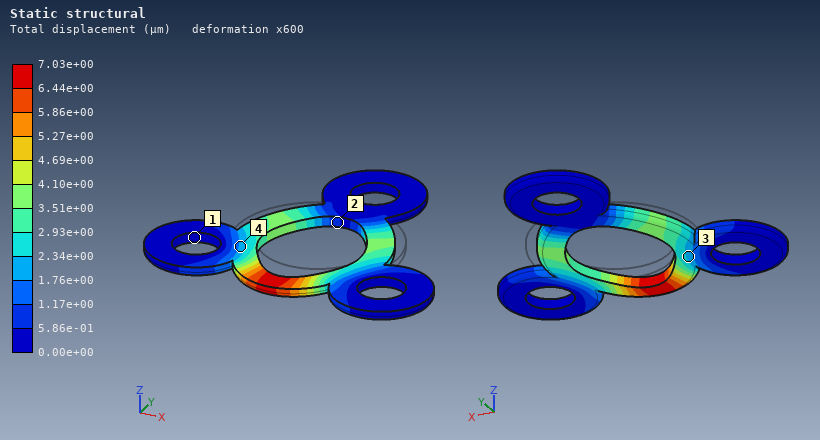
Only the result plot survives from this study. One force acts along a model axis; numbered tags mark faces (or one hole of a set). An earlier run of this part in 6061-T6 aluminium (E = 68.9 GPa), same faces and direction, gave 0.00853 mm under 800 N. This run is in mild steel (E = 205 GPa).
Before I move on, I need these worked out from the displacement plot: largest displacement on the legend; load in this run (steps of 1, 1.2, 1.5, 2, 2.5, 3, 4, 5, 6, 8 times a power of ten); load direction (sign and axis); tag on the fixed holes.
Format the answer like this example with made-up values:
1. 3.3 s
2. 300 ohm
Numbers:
1. 7.03e+00 µm
2. 2 kN
3. -Y
4. 1
